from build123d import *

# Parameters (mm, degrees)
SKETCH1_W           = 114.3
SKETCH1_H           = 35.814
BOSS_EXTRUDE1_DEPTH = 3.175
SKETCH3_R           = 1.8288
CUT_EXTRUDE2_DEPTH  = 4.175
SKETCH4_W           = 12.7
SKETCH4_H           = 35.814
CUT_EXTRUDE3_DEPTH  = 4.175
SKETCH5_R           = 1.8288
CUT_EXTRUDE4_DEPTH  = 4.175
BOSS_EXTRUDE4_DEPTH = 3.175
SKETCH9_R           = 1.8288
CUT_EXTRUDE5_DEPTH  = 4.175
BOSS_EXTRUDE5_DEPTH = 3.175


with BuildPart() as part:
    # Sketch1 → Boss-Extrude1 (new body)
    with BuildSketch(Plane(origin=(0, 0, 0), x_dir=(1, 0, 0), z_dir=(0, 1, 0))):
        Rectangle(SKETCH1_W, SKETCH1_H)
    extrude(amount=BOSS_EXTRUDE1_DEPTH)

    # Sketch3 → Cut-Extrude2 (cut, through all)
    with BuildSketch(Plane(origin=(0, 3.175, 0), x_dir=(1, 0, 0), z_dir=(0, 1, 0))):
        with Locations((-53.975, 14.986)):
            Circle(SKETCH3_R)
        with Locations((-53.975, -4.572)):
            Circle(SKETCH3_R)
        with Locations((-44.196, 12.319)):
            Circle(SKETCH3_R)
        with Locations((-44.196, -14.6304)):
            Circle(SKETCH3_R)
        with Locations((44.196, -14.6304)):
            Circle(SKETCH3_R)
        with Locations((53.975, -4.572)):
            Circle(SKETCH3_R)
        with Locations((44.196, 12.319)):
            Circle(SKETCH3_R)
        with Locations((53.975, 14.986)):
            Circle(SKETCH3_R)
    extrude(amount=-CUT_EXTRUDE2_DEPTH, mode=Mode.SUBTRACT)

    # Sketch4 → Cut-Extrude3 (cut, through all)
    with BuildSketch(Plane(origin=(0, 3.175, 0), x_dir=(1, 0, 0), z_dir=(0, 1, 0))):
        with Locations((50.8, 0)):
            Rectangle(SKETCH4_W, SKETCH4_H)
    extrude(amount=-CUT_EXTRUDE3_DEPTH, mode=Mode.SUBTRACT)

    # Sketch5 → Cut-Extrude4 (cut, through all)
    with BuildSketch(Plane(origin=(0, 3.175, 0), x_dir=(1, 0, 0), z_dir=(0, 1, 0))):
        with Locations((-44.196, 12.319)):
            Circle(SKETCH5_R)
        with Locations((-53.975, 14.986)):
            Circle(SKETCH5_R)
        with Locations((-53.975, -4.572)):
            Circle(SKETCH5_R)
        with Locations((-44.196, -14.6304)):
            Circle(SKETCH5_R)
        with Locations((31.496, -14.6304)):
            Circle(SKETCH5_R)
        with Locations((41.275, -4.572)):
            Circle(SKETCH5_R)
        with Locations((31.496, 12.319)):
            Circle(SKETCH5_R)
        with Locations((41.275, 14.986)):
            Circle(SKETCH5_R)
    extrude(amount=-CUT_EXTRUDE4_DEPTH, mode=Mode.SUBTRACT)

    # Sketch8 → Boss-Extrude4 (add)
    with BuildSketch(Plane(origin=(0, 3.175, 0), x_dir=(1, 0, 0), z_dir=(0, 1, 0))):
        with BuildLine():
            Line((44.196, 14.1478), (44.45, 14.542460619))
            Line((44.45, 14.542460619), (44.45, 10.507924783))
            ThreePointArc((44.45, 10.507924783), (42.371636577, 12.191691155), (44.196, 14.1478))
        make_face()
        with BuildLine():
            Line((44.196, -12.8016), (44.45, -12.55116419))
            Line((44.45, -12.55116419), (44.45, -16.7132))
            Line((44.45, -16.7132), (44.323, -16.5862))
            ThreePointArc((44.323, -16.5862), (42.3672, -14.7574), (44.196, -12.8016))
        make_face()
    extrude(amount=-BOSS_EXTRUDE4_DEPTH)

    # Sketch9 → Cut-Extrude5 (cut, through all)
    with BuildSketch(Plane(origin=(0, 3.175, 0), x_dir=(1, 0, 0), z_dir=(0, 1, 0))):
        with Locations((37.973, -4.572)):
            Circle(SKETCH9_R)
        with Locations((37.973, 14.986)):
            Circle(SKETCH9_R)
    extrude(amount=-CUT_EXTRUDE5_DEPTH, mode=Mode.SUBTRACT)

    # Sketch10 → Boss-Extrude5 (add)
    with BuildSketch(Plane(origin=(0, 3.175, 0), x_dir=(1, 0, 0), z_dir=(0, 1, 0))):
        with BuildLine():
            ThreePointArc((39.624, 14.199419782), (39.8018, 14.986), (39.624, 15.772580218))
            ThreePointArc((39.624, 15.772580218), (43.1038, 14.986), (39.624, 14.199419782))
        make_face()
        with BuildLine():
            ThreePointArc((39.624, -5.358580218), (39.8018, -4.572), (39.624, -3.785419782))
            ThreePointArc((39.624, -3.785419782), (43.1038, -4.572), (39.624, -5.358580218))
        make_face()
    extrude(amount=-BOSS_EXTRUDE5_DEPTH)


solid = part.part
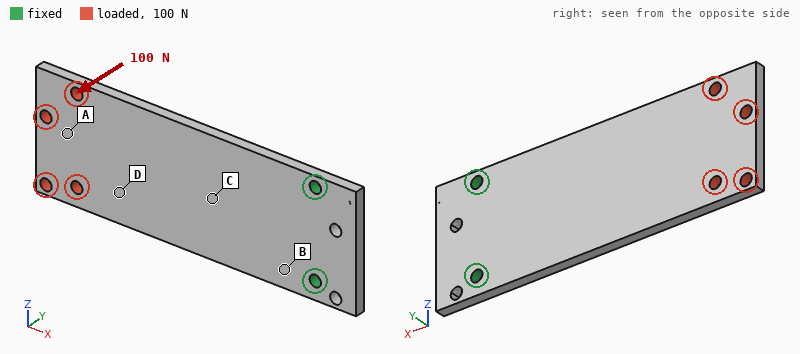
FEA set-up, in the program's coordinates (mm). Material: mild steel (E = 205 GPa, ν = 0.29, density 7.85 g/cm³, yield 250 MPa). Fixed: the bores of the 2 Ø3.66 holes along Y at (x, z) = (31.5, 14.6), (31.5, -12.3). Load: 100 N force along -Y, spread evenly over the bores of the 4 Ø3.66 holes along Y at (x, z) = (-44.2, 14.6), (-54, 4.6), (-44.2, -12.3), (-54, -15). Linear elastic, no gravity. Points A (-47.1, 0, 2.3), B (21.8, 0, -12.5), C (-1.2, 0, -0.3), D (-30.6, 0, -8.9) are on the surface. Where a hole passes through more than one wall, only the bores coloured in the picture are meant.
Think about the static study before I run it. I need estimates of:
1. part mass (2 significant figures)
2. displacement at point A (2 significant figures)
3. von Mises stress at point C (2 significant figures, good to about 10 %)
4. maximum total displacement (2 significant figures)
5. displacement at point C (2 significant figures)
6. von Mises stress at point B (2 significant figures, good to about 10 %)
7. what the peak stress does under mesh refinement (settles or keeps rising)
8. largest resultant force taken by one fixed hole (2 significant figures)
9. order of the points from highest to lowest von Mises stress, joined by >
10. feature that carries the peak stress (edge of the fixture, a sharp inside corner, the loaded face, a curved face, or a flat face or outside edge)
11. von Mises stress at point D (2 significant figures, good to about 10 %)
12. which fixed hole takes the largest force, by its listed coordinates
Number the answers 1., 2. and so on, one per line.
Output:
1. 89 g
2. 0.87 mm
3. 78 MPa
4. 1.0 mm
5. 0.20 mm
6. 120 MPa
7. keeps rising
8. 69 N
9. B > C > D > A
10. edge of the fixture
11. 32 MPa
12. (31.5, -12.3)
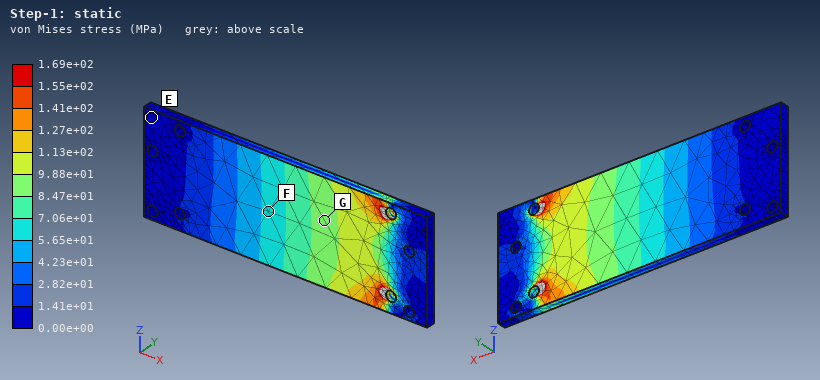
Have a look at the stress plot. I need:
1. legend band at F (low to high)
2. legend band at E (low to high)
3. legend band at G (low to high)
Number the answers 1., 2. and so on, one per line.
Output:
1. 5.65e+01 to 7.06e+01 MPa
2. 0.00e+00 to 1.41e+01 MPa
3. 8.47e+01 to 9.88e+01 MPa
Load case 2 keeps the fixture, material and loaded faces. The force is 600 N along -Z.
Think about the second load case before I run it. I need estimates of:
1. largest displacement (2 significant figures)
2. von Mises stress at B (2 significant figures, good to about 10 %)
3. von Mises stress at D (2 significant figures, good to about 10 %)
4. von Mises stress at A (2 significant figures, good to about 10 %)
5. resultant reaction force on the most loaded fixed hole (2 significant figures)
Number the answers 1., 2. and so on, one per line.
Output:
1. 58 µm
2. 46 MPa
3. 13 MPa
4. 9.4 MPa
5. 1.8 kN
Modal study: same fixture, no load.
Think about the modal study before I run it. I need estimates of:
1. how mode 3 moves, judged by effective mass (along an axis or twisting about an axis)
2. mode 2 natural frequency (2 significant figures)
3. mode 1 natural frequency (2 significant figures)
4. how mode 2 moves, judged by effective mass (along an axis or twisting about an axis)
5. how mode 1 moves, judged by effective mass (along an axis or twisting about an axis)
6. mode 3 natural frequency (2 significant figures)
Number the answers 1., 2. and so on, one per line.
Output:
1. along Y
2. 1800 Hz
3. 340 Hz
4. twisting about X
5. along Y
6. 2100 Hz
